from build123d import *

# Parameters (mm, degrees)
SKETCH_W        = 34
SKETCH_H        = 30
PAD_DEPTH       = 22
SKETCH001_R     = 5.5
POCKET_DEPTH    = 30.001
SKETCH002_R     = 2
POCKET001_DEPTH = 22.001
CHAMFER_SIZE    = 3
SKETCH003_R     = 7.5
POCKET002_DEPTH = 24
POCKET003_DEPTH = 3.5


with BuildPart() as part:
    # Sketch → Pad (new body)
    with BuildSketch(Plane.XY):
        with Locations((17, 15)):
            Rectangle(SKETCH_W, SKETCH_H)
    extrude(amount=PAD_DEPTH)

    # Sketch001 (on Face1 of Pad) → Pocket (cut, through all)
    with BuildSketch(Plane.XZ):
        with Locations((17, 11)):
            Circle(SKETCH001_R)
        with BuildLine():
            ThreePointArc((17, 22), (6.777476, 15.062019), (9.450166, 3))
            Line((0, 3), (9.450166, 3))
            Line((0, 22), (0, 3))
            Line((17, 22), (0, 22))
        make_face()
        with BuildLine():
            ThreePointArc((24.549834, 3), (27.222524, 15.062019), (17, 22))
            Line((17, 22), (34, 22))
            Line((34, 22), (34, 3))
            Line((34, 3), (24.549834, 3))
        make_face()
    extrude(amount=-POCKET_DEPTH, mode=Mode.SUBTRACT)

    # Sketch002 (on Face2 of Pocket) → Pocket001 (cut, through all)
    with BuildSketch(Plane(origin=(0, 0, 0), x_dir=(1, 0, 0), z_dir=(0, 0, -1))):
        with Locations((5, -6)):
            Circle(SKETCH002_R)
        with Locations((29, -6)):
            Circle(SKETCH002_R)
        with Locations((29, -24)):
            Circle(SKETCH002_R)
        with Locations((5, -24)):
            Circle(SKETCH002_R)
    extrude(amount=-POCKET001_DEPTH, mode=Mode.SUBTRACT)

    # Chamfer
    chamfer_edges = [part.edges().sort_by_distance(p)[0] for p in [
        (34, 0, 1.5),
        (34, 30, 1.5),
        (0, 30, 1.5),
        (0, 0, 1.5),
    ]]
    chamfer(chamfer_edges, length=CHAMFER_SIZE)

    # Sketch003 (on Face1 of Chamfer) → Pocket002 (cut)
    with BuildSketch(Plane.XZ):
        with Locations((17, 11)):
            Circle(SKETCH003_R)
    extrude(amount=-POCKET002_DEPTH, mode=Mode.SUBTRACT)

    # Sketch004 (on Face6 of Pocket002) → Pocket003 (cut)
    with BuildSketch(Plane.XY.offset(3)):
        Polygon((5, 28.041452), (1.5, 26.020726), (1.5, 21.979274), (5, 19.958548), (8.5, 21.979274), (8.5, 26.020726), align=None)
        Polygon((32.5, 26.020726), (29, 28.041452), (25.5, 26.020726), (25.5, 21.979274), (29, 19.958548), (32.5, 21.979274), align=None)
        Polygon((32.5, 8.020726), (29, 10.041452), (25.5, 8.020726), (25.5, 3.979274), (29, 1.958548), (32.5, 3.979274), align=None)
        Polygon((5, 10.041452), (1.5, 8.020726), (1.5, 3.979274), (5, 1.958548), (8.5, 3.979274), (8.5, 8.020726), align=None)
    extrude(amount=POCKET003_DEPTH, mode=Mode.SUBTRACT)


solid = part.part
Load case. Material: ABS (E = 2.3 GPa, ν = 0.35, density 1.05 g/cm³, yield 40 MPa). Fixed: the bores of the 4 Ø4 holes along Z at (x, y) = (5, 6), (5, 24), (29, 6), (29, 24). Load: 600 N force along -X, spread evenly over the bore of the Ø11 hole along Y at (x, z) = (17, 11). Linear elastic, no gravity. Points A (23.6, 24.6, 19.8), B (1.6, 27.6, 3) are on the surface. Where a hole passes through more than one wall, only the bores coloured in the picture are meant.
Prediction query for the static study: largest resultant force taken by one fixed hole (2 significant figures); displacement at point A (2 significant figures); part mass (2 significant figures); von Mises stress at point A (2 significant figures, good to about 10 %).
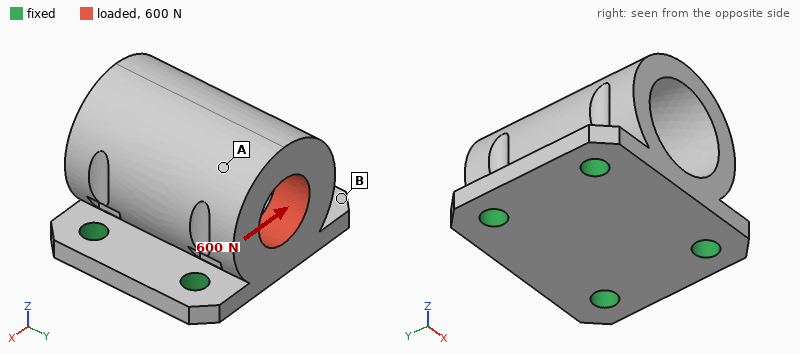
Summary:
320 N
0.33 mm
8.8 g
5.9 MPa
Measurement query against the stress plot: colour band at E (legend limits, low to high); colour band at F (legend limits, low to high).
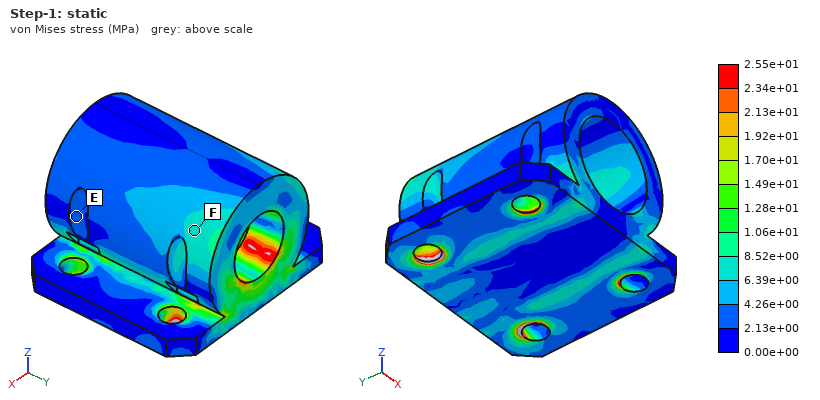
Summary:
2.13e+00 to 4.26e+00 MPa
6.39e+00 to 8.52e+00 MPa
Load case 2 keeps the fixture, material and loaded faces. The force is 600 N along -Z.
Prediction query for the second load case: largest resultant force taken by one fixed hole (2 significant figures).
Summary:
340 N
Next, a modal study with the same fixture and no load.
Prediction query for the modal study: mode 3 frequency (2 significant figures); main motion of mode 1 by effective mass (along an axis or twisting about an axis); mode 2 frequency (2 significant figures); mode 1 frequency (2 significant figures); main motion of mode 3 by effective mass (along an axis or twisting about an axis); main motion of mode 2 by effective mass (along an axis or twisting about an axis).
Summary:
5600 Hz
along X
3400 Hz
2800 Hz
along Z
along Y
